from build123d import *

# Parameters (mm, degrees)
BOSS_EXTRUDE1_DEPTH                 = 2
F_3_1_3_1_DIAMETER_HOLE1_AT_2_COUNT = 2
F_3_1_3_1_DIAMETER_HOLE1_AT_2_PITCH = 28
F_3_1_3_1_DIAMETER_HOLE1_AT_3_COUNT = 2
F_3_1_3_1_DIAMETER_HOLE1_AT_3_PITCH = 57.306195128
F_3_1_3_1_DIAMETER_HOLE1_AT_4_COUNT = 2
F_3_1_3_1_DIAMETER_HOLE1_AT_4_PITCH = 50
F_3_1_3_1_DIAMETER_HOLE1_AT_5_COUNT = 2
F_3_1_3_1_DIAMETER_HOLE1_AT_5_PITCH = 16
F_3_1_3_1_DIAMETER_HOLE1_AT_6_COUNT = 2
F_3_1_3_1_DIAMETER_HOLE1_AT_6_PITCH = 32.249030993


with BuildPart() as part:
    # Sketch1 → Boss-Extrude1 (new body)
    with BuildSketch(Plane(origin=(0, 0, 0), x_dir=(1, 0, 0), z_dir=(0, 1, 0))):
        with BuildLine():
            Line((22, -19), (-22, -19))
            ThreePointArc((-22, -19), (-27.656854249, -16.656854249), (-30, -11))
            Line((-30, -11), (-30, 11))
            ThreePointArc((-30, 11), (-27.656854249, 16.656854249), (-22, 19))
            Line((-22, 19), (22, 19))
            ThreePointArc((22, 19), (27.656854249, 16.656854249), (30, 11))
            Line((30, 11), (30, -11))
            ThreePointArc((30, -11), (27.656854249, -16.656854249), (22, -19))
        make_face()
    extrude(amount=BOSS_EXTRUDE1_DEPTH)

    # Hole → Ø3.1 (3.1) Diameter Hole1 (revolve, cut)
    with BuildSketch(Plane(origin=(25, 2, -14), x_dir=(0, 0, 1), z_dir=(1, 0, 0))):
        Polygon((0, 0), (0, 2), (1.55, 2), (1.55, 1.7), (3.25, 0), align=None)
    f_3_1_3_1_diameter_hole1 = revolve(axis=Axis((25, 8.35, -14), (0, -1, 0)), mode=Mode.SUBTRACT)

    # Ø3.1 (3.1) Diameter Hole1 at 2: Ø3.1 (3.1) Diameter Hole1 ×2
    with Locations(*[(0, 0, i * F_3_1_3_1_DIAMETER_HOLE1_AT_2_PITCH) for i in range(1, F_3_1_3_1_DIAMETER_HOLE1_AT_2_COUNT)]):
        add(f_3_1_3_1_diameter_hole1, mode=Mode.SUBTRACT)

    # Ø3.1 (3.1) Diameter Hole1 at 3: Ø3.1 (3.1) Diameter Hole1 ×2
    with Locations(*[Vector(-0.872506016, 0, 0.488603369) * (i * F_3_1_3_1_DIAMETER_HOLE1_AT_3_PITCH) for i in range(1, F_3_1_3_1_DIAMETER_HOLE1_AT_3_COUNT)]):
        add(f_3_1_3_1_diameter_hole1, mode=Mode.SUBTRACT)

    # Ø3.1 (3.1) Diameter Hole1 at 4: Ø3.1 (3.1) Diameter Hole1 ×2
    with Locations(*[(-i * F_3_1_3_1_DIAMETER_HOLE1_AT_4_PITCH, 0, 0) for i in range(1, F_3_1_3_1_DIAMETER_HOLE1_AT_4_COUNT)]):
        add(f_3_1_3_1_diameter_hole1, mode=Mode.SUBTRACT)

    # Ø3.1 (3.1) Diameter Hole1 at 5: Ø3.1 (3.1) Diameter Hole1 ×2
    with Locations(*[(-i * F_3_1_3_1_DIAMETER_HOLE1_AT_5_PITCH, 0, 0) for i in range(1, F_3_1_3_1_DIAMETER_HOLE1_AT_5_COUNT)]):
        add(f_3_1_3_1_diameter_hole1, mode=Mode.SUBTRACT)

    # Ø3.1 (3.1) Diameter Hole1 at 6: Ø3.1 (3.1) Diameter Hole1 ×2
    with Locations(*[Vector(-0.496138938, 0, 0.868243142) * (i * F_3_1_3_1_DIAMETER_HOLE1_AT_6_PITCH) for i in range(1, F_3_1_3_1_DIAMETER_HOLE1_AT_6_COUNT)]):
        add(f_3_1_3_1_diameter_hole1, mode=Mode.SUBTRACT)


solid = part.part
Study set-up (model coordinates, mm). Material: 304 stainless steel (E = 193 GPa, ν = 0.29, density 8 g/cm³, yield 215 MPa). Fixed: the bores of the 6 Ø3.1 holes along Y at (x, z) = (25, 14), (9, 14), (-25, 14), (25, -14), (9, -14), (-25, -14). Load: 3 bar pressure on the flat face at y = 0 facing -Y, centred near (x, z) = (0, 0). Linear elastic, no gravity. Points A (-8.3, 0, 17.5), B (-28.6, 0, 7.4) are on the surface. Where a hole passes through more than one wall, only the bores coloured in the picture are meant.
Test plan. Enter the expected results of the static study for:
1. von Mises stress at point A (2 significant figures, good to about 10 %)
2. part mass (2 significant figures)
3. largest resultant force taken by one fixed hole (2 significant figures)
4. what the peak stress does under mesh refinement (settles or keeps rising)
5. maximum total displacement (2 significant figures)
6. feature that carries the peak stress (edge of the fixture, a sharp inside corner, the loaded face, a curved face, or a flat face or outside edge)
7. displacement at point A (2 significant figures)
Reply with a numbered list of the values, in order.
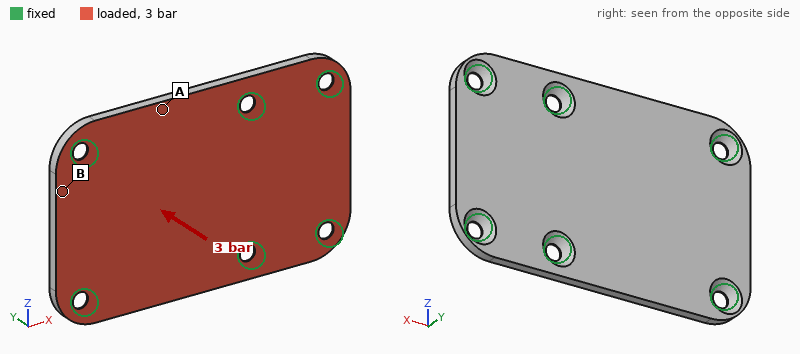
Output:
1. 27 MPa
2. 34 g
3. 270 N
4. keeps rising
5. 19 µm
6. edge of the fixture
7. 13 µm
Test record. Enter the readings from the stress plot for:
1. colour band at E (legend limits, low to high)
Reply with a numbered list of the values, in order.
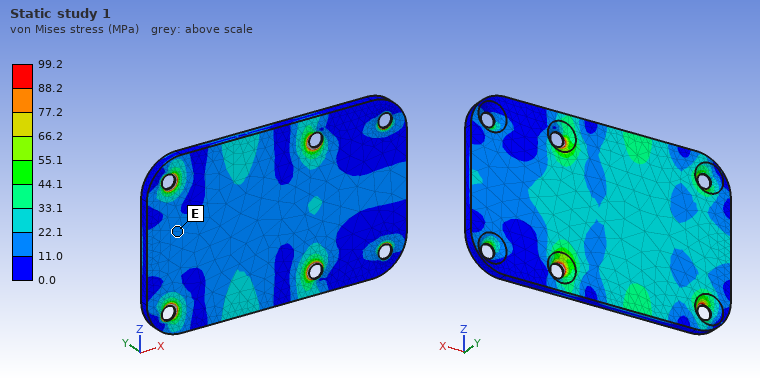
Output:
1. 11.0 to 22.1 MPa
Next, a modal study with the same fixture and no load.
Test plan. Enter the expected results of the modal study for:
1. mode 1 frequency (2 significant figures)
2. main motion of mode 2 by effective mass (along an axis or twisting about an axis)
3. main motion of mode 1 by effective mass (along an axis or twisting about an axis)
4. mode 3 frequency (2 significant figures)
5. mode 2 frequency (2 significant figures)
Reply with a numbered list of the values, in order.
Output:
1. 6000 Hz
2. twisting about X
3. along Y
4. 9700 Hz
5. 8500 Hz
